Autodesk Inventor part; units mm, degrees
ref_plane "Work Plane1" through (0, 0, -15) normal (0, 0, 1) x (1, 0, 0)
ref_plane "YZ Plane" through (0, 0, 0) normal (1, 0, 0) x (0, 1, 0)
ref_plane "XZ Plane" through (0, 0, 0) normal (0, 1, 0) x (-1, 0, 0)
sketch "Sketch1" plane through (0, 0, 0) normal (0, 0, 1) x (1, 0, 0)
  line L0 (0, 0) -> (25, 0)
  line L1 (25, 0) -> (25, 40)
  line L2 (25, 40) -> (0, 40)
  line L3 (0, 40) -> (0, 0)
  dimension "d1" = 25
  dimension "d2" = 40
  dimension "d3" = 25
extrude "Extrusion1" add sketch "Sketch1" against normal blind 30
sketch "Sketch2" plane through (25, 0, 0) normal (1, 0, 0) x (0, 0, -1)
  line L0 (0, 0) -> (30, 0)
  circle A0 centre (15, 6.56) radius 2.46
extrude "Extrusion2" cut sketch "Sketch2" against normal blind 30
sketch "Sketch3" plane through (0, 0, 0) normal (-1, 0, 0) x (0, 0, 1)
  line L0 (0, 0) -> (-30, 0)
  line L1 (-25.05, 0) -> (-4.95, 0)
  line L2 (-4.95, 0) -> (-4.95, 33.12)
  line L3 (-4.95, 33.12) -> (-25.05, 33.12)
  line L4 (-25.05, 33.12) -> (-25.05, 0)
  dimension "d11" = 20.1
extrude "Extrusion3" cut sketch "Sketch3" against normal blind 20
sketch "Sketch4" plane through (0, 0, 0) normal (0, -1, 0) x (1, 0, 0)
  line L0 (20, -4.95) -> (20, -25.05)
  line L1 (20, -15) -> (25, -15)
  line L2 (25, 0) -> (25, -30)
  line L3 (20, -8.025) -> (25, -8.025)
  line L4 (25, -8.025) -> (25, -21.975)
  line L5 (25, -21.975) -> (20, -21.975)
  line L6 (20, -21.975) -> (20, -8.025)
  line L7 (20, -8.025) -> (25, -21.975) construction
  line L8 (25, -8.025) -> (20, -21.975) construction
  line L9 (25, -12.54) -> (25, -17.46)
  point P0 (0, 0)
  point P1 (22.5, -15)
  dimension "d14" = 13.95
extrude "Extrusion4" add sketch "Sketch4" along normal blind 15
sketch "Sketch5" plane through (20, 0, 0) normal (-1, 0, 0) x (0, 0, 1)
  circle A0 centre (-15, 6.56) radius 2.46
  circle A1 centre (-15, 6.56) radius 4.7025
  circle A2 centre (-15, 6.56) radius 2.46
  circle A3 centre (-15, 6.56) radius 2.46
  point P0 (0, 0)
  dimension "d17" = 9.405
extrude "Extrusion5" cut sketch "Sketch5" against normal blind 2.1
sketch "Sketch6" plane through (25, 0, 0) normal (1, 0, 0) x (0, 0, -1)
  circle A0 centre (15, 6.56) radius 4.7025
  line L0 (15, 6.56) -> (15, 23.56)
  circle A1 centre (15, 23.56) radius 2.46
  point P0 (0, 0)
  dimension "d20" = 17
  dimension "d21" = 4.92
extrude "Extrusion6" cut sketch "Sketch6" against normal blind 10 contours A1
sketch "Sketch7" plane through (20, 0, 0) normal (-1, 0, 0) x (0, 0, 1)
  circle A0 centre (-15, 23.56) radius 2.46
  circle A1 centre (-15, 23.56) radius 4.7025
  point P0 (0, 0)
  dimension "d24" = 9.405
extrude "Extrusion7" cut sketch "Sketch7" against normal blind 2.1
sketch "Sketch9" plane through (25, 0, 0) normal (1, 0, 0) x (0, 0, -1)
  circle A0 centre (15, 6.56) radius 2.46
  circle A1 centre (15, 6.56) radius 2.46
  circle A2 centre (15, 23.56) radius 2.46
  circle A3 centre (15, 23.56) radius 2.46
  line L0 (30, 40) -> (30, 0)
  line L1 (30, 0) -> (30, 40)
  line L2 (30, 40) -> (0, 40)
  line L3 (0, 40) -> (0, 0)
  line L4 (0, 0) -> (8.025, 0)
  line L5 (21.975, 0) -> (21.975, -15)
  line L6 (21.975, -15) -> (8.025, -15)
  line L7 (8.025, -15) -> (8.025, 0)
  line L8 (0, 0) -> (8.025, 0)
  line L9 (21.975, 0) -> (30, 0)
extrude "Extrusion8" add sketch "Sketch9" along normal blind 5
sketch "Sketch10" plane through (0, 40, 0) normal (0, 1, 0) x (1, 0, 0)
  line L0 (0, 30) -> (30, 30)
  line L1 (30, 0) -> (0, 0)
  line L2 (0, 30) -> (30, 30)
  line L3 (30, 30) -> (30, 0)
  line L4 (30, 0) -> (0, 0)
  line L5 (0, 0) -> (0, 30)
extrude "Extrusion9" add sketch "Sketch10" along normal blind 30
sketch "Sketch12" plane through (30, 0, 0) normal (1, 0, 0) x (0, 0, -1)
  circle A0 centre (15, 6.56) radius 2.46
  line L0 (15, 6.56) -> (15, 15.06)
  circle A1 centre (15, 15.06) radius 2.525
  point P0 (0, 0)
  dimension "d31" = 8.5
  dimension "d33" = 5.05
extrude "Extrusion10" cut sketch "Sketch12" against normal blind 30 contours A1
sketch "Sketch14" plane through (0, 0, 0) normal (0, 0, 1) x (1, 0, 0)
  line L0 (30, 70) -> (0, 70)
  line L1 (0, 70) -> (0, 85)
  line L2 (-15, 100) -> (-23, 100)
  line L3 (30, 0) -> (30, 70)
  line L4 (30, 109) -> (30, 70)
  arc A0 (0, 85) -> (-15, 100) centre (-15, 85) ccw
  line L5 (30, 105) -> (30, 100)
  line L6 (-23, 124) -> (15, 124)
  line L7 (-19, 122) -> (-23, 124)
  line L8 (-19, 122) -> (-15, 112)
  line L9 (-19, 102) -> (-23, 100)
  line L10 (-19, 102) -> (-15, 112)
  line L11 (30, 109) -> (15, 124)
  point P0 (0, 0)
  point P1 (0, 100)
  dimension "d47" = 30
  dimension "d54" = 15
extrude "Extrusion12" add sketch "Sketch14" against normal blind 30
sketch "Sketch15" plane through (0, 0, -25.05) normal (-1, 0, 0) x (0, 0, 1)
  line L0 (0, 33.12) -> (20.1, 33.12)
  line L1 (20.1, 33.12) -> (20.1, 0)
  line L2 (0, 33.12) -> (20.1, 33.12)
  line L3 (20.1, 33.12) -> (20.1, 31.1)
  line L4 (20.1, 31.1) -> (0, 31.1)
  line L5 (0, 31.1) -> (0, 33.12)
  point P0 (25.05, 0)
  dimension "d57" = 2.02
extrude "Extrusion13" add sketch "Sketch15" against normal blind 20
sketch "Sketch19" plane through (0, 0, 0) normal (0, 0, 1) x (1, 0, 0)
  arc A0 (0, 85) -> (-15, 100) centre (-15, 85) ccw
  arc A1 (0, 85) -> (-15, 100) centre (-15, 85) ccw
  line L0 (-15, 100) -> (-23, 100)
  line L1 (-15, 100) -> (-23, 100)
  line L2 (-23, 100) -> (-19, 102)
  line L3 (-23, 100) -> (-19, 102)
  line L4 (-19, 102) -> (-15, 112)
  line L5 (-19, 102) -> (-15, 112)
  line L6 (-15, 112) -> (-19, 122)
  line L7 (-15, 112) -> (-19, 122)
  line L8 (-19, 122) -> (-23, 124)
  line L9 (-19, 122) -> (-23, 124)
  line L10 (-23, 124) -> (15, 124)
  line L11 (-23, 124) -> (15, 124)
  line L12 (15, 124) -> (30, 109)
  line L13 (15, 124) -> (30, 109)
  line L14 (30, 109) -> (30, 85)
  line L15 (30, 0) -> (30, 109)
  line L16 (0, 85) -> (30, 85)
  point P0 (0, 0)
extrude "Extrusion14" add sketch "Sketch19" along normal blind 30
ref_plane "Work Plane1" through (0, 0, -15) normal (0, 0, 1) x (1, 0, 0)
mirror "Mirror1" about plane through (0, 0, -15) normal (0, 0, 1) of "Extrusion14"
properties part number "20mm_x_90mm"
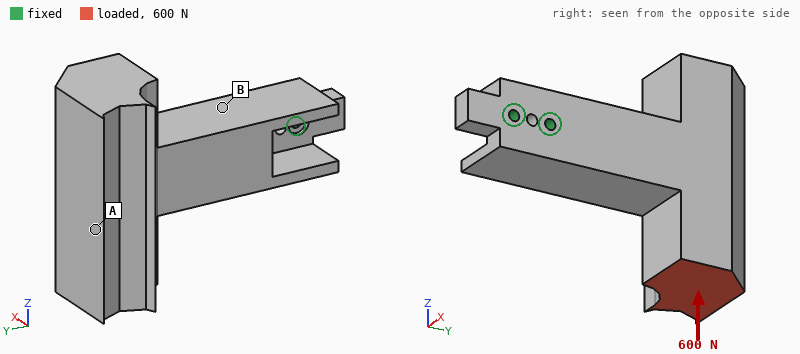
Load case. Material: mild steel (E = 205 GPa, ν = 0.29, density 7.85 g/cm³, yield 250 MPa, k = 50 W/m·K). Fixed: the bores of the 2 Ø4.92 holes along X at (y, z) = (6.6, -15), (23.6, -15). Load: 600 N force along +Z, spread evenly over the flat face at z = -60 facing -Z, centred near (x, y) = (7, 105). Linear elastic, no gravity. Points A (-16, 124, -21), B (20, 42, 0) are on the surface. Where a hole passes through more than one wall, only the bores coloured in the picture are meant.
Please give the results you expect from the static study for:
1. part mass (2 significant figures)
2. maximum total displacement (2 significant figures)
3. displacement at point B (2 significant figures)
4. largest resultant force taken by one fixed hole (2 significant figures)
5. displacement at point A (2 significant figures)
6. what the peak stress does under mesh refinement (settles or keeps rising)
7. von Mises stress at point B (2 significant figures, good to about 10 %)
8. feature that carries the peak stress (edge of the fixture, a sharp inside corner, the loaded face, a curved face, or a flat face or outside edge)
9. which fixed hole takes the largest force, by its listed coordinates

1.6 kg
42 µm
6.8 µm
2.7 kN
37 µm
keeps rising
10 MPa
edge of the fixture
(23.6, -15)
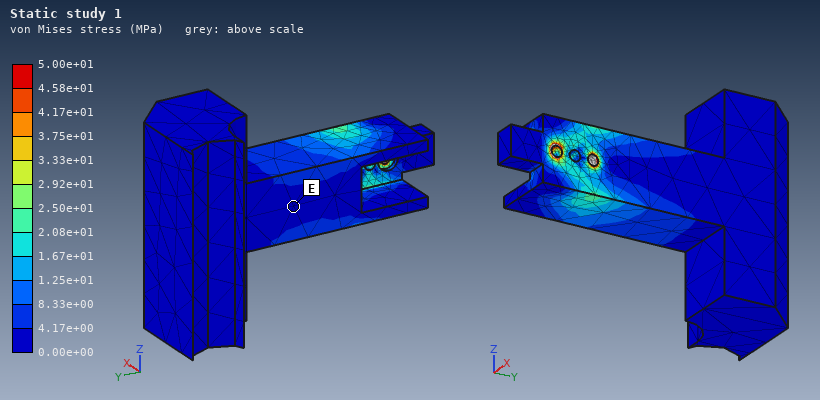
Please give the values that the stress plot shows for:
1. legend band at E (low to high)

0.00e+00 to 4.17e+00 MPa
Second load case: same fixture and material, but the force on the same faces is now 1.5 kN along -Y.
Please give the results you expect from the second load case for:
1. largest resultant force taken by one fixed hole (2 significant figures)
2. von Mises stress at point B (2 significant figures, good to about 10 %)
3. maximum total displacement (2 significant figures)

3.2 kN
19 MPa
72 µm
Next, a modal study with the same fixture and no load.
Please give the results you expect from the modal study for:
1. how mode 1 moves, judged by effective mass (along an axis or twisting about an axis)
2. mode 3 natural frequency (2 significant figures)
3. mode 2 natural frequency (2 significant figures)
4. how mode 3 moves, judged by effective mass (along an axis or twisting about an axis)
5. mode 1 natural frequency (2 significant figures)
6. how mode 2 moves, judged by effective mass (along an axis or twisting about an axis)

along X
1100 Hz
640 Hz
twisting about Y
570 Hz
along Z
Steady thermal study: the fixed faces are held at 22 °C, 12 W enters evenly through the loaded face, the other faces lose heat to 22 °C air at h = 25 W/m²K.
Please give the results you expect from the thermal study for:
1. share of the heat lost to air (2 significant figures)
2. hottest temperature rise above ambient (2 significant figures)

57 %
18 K
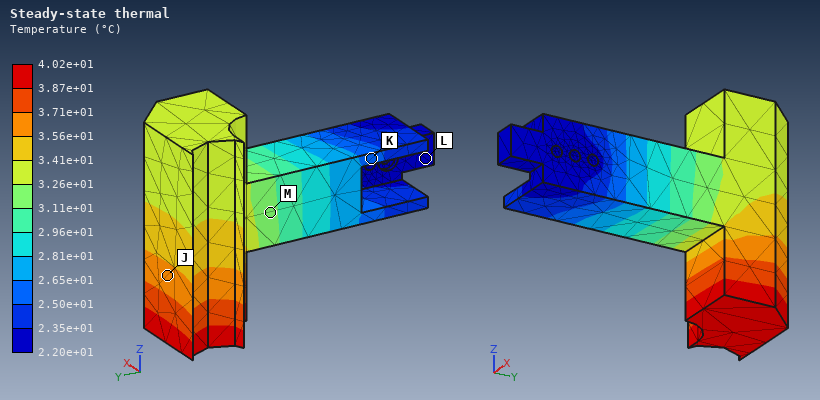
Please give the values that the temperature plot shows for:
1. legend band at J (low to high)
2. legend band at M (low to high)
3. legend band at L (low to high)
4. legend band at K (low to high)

3.56e+01 to 3.71e+01 °C
3.11e+01 to 3.26e+01 °C
2.20e+01 to 2.35e+01 °C
2.50e+01 to 2.65e+01 °C
